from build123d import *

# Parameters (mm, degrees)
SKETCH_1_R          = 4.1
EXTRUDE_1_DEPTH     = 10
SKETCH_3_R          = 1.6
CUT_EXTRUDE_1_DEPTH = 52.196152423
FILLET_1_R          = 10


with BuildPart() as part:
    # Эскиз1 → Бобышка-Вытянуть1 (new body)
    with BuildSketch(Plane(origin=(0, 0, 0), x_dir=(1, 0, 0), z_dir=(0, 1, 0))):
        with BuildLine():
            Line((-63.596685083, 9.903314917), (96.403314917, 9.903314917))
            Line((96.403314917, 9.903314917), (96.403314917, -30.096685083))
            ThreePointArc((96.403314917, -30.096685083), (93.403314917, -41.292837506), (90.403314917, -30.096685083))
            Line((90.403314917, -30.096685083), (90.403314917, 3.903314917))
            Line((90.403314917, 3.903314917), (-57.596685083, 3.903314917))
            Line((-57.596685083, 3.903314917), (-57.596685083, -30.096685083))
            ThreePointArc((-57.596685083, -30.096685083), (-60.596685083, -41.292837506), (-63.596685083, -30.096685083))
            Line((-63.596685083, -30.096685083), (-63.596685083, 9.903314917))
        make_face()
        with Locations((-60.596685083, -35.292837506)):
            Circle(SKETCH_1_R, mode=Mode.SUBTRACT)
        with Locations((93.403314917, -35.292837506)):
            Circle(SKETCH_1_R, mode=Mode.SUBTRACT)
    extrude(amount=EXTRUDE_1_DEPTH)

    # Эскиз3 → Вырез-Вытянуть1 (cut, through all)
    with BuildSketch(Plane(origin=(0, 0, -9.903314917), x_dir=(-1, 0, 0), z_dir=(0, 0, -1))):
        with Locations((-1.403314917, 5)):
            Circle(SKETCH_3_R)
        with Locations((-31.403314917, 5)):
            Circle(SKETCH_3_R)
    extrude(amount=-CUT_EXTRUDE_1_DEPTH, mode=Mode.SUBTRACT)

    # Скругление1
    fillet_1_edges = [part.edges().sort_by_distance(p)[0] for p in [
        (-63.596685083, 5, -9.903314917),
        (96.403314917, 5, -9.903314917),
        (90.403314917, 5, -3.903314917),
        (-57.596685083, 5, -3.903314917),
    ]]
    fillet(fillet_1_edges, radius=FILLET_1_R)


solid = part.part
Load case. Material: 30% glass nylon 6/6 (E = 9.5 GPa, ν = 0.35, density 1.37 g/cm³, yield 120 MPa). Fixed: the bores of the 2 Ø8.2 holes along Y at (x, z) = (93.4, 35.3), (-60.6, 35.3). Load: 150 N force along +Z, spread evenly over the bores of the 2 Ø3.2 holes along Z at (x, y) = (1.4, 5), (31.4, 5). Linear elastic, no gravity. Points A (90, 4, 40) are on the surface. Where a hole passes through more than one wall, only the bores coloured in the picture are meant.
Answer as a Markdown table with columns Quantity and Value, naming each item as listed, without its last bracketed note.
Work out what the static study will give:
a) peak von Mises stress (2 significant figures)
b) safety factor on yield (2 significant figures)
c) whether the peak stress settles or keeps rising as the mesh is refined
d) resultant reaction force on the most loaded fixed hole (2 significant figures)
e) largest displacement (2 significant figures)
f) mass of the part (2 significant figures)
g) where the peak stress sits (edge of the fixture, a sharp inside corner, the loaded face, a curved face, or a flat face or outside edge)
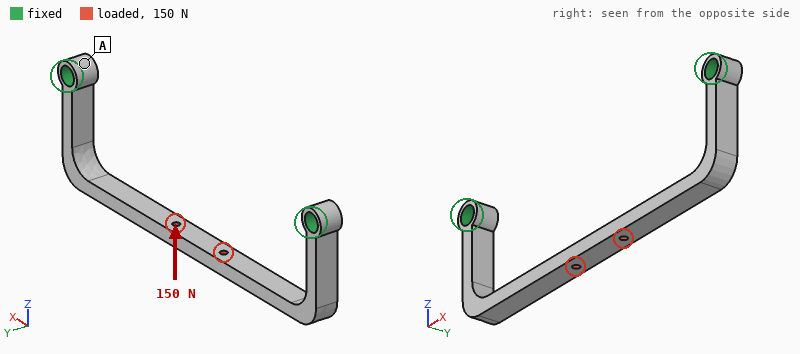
| Quantity | Value |
|---|---|
| peak von Mises stress | 81 MPa |
| safety factor on yield | 1.5 |
| whether the peak stress settles or keeps rising as the mesh is refined | settles |
| resultant reaction force on the most loaded fixed hole | 130 N |
| largest displacement | 1.6 mm |
| mass of the part | 20 g |
| where the peak stress sits | the loaded face |
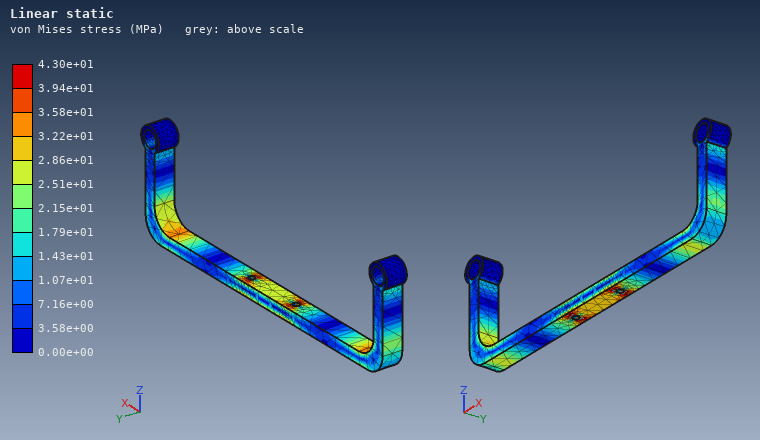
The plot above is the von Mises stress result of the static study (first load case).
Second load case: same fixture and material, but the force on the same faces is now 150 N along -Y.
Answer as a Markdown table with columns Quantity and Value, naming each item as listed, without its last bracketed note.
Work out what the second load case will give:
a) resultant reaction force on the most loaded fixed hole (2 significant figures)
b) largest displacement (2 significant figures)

| Quantity | Value |
|---|---|
| resultant reaction force on the most loaded fixed hole | 75 N |
| largest displacement | 1.8 mm |
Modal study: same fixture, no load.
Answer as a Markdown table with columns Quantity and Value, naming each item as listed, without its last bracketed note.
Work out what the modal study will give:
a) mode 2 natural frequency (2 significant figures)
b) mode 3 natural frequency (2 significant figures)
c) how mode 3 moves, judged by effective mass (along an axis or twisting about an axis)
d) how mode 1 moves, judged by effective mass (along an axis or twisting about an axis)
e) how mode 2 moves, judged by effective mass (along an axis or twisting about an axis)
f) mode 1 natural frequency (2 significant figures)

| Quantity | Value |
|---|---|
| mode 2 natural frequency | 670 Hz |
| mode 3 natural frequency | 760 Hz |
| how mode 3 moves, judged by effective mass | along X |
| how mode 1 moves, judged by effective mass | along Y |
| how mode 2 moves, judged by effective mass | along Z |
| mode 1 natural frequency | 550 Hz |
